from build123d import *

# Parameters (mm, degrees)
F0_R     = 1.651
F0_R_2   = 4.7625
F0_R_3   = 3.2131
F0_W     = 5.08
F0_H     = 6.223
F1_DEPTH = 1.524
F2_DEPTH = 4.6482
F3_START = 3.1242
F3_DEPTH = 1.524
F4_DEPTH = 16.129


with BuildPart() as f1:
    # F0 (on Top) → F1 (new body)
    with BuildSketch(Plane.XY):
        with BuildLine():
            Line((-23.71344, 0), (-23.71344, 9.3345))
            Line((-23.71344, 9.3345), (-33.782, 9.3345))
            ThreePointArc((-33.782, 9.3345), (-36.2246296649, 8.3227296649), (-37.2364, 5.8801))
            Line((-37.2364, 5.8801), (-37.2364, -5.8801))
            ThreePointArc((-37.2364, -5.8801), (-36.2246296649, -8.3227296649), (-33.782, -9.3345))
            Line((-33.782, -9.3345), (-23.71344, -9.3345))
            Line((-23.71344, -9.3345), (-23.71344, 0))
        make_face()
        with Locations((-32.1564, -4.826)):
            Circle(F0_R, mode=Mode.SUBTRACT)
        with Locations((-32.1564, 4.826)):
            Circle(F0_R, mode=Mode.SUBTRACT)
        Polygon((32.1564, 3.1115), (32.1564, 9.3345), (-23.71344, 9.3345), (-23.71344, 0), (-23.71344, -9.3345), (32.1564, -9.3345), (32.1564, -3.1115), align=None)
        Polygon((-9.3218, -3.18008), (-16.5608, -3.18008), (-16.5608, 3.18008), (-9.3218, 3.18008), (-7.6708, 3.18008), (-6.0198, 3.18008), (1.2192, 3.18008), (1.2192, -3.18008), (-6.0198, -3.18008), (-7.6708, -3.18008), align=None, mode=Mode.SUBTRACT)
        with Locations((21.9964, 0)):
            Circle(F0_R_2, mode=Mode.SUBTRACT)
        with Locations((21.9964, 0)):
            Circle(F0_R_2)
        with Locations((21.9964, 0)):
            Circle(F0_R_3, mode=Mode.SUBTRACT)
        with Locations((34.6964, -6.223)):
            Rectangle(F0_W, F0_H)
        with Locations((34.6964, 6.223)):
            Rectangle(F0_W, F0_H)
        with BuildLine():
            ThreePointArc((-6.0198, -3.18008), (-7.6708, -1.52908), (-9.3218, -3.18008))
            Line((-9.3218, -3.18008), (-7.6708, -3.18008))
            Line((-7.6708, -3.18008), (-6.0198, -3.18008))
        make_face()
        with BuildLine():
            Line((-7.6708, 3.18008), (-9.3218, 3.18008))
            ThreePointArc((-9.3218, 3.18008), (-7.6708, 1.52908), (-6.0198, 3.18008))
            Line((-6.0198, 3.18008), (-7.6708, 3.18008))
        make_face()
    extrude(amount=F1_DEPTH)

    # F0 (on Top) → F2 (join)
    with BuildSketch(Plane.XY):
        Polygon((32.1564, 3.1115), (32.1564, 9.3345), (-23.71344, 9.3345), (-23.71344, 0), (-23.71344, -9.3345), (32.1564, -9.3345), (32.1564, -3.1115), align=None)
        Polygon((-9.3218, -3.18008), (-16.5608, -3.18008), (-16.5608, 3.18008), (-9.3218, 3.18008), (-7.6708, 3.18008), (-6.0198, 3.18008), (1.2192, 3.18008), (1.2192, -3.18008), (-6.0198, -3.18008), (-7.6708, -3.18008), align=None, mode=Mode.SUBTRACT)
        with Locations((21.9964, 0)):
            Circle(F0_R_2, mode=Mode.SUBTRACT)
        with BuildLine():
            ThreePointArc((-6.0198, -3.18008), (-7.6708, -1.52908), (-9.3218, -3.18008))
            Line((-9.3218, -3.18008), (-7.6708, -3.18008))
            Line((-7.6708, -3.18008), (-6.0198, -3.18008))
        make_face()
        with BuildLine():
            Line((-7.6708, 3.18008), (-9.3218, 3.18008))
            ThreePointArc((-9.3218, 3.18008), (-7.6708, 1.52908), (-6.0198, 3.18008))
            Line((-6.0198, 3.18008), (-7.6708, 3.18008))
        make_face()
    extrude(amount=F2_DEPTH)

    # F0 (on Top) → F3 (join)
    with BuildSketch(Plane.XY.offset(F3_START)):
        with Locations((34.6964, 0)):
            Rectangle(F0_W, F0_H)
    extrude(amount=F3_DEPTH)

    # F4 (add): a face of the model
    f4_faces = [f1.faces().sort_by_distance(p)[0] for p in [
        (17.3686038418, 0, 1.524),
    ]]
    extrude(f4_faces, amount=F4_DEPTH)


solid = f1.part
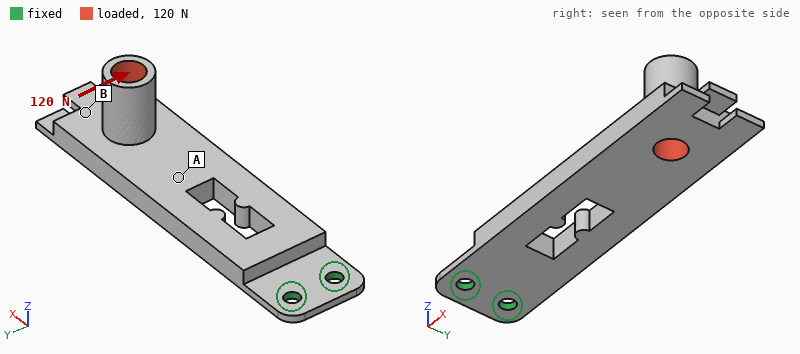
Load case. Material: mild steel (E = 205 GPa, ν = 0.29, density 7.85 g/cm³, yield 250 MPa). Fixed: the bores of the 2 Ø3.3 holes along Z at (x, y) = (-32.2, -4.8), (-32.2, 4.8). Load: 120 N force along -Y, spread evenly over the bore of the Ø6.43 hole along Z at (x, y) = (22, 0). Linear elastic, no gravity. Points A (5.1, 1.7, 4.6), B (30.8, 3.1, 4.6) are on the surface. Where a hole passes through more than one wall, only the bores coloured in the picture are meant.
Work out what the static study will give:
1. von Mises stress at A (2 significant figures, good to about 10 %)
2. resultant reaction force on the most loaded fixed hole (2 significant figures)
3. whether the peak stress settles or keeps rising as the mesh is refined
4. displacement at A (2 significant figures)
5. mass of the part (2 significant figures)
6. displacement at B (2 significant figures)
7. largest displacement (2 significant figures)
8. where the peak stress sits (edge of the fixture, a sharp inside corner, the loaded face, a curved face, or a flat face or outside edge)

23 MPa
560 N
keeps rising
26 µm
41 g
42 µm
68 µm
edge of the fixture
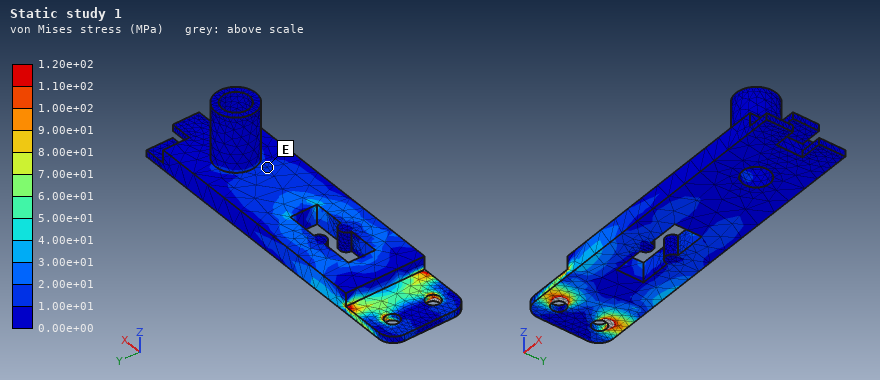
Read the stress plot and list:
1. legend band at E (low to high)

1.00e+01 to 2.00e+01 MPa
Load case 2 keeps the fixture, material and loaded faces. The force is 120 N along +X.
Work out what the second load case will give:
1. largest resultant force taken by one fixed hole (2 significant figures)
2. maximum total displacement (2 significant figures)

61 N
0.48 mm
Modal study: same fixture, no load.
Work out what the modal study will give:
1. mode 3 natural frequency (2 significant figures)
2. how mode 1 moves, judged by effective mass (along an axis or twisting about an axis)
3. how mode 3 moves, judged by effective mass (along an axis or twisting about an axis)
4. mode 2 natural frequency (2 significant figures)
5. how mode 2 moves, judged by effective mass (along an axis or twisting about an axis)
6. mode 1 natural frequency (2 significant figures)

2700 Hz
along Z
twisting about X
2000 Hz
along Y
250 Hz
